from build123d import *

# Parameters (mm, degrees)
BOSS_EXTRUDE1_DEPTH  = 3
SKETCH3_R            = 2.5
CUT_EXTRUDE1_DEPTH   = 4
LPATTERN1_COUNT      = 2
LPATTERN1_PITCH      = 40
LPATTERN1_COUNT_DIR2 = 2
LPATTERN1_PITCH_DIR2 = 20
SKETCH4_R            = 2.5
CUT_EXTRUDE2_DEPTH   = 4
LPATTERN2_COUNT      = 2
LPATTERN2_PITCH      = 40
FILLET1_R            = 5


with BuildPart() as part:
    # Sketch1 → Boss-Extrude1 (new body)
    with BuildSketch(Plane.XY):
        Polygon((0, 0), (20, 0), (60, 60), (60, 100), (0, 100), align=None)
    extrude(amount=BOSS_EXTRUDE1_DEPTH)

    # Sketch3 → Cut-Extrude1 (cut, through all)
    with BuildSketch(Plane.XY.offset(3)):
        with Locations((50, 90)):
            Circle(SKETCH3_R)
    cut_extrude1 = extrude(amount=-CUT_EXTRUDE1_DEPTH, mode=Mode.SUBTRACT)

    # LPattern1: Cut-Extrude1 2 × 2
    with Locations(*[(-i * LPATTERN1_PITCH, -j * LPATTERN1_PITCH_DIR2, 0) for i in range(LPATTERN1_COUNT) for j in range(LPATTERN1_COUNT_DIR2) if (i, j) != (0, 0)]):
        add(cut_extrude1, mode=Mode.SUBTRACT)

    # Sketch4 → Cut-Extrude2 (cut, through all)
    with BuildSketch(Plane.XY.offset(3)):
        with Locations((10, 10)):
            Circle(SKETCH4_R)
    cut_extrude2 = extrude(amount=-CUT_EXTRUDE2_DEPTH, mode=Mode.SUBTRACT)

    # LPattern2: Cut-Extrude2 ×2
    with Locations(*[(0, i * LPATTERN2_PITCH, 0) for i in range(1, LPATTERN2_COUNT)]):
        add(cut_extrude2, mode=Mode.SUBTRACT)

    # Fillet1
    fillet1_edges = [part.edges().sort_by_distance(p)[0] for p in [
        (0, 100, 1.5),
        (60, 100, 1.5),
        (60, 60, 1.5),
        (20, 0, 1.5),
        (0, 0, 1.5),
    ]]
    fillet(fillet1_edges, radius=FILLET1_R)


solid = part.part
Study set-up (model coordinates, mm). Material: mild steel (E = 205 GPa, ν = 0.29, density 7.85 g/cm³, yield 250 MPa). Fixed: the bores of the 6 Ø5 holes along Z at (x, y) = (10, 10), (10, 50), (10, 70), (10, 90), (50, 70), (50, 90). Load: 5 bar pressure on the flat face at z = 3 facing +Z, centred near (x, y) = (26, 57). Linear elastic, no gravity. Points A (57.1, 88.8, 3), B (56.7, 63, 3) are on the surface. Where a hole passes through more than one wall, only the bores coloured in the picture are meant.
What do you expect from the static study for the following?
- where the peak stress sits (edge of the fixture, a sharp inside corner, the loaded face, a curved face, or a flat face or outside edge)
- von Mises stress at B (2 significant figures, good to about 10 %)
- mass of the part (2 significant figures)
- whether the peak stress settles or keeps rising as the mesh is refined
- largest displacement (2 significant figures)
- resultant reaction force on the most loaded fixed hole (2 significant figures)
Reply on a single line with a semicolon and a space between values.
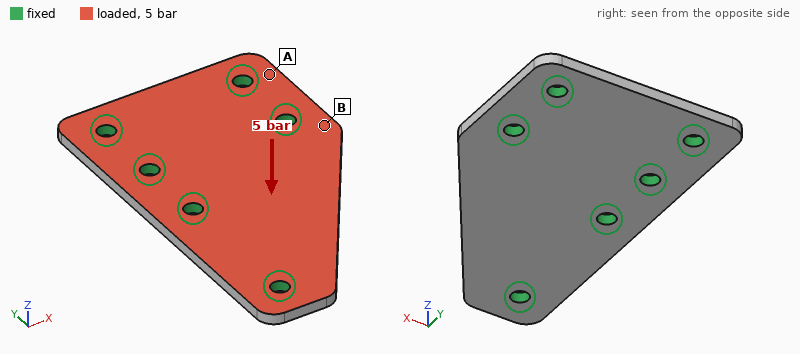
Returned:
edge of the fixture; 49 MPa; 110 g; keeps rising; 63 µm; 540 N
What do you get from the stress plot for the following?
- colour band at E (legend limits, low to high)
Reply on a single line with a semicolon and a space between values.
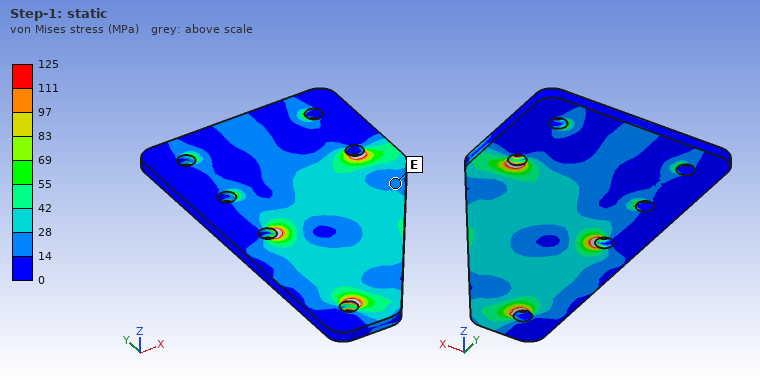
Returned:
14 to 28 MPa
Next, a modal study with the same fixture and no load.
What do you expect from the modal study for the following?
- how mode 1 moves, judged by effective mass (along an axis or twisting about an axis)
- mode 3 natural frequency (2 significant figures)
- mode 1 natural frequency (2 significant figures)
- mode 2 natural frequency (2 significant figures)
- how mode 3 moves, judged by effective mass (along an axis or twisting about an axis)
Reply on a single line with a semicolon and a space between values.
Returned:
along Z; 10 kHz; 4000 Hz; 8500 Hz; along Z
